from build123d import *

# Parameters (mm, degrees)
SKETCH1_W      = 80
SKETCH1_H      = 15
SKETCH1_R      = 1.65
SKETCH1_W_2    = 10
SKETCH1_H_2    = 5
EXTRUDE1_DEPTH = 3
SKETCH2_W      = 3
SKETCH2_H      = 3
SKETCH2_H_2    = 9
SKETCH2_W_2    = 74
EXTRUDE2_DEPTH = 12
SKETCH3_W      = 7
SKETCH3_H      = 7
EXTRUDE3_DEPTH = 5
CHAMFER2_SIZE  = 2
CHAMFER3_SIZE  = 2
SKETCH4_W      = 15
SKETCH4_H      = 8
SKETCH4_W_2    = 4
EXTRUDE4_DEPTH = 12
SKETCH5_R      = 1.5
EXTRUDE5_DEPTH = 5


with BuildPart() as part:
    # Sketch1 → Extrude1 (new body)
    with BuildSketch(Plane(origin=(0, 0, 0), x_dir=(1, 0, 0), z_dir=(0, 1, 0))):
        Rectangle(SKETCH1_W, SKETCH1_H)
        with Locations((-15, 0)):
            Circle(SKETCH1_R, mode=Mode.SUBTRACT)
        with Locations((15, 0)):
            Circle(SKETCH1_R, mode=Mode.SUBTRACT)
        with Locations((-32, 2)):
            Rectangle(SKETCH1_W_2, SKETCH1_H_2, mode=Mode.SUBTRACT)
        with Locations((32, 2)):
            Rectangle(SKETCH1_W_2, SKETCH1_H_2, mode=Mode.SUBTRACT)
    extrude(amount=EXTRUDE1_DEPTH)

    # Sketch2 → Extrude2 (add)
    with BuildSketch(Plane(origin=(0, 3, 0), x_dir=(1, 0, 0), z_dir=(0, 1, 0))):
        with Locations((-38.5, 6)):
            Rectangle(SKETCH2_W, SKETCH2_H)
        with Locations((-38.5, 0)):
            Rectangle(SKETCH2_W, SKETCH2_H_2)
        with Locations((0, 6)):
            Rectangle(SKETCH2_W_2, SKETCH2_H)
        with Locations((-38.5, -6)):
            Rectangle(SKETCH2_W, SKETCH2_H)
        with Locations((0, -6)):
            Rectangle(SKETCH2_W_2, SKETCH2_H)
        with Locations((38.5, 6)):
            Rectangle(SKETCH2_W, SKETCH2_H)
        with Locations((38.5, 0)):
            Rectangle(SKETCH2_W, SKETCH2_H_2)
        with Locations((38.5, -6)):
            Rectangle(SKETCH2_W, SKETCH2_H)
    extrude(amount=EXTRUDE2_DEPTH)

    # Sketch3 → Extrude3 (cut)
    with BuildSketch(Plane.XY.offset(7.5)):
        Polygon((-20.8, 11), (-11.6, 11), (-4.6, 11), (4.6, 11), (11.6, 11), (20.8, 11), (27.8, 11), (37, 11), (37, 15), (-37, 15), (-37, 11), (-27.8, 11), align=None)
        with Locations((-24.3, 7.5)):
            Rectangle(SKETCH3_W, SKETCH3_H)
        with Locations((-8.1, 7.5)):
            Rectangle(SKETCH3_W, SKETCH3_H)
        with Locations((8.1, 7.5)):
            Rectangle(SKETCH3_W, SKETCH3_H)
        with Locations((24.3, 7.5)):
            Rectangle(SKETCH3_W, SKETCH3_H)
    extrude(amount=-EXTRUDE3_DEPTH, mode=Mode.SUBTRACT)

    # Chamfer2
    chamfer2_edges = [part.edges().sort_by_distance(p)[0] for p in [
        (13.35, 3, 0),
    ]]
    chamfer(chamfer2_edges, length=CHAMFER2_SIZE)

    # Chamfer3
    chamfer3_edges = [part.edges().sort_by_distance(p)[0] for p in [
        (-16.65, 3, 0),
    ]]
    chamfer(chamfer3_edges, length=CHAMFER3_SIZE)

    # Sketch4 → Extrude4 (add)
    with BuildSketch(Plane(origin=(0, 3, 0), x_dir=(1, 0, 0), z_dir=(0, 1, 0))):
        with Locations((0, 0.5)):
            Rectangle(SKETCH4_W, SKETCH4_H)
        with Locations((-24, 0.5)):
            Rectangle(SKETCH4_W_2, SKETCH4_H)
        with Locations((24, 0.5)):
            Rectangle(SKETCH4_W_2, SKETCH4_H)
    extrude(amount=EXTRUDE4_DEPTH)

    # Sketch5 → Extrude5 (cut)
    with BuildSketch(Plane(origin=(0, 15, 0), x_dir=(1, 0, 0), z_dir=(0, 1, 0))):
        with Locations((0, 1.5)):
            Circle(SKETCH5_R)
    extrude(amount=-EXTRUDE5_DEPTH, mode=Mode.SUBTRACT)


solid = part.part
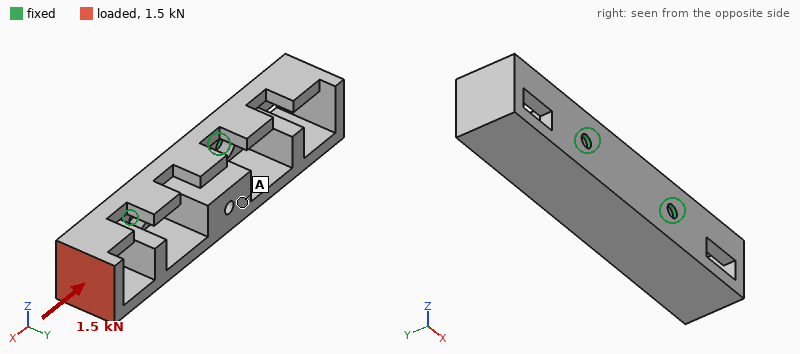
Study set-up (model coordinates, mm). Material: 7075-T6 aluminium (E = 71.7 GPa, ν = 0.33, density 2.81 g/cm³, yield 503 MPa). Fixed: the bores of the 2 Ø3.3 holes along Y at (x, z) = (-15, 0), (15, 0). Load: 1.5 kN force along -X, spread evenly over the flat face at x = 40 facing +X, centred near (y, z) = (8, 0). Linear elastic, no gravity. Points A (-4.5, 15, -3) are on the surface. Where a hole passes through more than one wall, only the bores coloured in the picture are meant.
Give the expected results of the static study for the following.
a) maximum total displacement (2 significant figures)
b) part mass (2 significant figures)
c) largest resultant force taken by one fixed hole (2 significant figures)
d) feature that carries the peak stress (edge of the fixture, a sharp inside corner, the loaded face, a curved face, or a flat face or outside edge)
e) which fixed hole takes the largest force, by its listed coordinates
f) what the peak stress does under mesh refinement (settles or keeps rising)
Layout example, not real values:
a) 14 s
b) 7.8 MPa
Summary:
a) 0.12 mm
b) 29 g
c) 910 N
d) edge of the fixture
e) (15, 0)
f) keeps rising
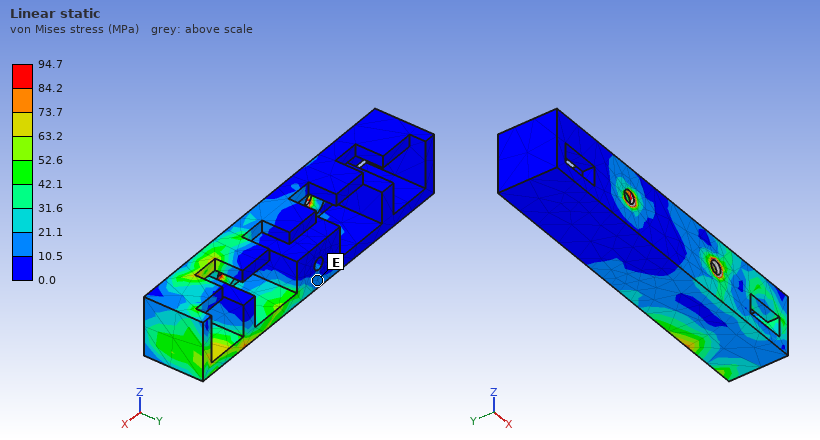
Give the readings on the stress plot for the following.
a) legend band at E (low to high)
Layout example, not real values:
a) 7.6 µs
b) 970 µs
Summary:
a) 10.5 to 21.1 MPa
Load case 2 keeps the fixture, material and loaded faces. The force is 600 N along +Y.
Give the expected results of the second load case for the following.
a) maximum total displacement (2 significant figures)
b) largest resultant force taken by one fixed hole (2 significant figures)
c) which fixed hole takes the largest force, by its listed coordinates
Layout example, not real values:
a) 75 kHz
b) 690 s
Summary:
a) 0.17 mm
b) 1.2 kN
c) (15, 0)
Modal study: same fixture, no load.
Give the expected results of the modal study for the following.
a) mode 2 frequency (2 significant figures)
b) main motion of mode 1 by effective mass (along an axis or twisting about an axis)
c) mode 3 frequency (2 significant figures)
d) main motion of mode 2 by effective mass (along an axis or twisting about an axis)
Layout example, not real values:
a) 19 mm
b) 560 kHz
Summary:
a) 4700 Hz
b) along Z
c) 5600 Hz
d) twisting about Y
